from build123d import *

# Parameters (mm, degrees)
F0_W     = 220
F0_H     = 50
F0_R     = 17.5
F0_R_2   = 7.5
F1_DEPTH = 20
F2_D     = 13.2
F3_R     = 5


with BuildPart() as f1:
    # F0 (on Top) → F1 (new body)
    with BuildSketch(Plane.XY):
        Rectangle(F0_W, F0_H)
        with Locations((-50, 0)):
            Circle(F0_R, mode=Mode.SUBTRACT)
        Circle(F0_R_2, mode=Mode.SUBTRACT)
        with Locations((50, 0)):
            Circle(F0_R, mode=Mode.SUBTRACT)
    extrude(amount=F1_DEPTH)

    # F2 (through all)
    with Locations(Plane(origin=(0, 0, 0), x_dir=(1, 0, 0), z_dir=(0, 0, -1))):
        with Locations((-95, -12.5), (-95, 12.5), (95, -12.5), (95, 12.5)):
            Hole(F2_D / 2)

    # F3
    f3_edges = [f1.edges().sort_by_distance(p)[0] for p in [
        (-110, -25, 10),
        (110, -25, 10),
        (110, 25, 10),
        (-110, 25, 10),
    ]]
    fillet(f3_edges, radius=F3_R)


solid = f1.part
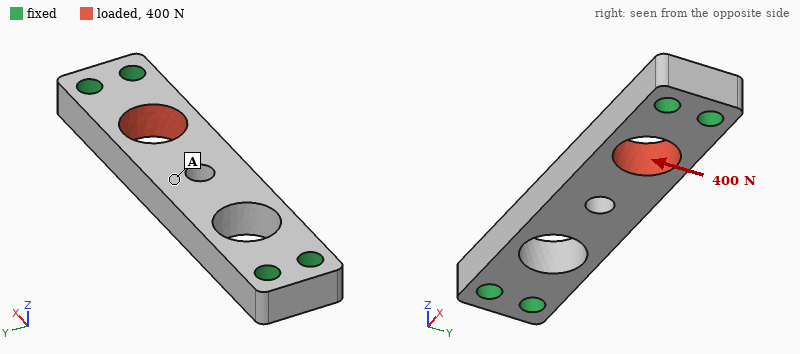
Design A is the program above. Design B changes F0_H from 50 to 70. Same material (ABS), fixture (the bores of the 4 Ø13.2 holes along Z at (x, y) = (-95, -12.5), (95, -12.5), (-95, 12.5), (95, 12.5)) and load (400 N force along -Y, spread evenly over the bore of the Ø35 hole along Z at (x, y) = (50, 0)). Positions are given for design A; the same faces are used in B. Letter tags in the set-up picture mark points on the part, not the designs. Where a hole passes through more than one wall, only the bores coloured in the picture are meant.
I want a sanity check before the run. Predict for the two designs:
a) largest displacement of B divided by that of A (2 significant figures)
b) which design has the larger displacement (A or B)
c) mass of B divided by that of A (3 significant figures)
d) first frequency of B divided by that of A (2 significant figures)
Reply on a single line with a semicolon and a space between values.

0.40; A; 1.53; 0.99
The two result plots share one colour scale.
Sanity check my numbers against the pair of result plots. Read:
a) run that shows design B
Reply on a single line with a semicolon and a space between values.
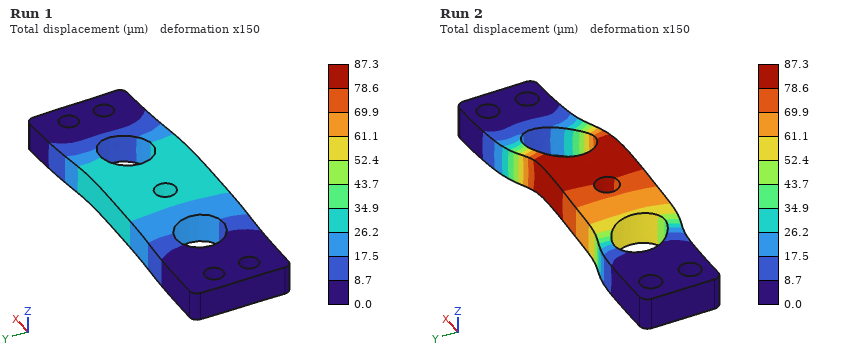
Run 1
